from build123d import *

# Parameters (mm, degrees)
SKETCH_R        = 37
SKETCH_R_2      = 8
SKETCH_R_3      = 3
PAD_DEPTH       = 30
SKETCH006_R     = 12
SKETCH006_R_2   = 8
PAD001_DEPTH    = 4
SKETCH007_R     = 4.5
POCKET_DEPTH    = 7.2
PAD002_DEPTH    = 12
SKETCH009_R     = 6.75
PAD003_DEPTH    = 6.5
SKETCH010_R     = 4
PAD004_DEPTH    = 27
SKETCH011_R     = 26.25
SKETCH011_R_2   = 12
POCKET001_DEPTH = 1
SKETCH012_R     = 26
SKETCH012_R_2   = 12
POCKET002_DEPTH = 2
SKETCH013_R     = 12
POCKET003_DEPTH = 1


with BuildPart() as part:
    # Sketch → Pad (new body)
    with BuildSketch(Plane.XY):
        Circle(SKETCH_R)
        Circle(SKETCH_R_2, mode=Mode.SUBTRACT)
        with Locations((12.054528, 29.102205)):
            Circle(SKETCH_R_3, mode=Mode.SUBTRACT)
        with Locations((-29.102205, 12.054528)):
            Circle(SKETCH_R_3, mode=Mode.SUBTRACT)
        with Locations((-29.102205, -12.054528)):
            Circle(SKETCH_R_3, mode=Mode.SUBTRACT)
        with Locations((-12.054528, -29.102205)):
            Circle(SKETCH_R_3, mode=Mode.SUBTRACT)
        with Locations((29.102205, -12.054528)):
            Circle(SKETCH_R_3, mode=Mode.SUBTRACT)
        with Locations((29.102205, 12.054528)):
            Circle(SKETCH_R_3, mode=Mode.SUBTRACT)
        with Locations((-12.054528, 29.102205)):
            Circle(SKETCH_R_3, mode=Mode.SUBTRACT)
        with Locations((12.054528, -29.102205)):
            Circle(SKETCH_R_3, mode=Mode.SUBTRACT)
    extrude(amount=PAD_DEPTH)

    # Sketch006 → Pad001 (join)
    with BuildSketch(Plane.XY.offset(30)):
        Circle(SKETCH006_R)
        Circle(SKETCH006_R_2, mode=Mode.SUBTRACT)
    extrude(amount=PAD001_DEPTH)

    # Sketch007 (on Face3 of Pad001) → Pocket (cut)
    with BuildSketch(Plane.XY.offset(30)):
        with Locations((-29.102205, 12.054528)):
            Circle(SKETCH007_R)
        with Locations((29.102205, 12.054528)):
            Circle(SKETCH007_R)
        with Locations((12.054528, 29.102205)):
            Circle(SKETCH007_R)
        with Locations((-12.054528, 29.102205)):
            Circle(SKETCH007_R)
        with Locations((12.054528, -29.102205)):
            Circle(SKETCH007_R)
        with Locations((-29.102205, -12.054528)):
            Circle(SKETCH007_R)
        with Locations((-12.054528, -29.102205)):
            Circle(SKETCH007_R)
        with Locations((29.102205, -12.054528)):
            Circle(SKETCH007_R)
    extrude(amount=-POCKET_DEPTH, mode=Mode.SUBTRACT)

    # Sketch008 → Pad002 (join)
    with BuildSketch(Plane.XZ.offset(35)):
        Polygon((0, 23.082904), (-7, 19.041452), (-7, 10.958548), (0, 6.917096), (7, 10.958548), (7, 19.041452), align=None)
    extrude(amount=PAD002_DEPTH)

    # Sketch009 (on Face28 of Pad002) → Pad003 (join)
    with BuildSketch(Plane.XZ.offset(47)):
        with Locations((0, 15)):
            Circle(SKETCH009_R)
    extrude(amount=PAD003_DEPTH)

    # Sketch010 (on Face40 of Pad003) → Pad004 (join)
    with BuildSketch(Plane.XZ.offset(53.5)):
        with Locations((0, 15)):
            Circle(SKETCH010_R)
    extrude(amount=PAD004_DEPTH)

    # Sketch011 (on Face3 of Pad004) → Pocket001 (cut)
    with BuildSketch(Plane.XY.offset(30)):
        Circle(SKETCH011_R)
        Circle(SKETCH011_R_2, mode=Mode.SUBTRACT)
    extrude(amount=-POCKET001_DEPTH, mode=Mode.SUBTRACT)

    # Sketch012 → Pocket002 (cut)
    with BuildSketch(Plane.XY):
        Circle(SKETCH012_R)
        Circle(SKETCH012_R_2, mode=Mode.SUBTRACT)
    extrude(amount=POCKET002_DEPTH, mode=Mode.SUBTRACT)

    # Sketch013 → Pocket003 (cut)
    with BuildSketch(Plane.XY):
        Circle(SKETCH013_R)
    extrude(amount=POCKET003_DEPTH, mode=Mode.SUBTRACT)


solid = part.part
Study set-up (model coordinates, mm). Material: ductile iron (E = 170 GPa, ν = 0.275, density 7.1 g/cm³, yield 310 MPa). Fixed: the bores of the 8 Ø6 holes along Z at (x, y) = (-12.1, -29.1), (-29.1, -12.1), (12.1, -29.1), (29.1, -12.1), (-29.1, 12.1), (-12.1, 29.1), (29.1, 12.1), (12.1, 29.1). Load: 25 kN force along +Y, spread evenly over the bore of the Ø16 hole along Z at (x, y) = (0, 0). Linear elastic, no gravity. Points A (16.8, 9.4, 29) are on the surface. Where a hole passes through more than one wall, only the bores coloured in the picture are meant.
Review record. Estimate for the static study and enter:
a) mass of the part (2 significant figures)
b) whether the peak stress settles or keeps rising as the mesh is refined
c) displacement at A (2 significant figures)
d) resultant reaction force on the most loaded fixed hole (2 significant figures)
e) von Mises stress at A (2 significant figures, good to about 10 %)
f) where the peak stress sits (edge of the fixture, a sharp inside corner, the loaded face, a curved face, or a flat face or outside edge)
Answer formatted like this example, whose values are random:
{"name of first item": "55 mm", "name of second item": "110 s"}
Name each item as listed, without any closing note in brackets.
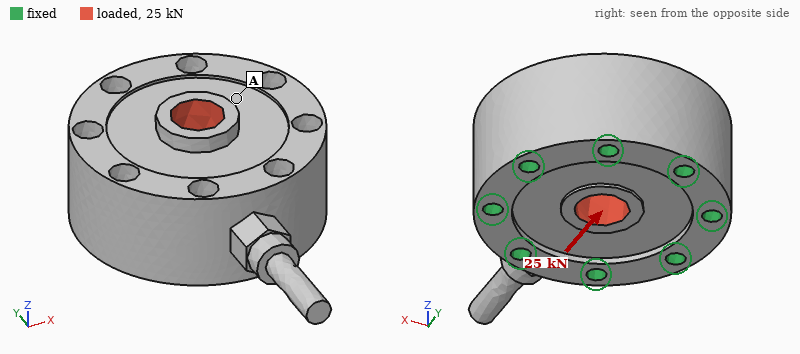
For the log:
{"mass of the part": "810 g", "whether the peak stress settles or keeps rising as the mesh is refined": "keeps rising", "displacement at A": "1.00 µm", "resultant reaction force on the most loaded fixed hole": "4.8 kN", "von Mises stress at A": "7.8 MPa", "where the peak stress sits": "edge of the fixture"}
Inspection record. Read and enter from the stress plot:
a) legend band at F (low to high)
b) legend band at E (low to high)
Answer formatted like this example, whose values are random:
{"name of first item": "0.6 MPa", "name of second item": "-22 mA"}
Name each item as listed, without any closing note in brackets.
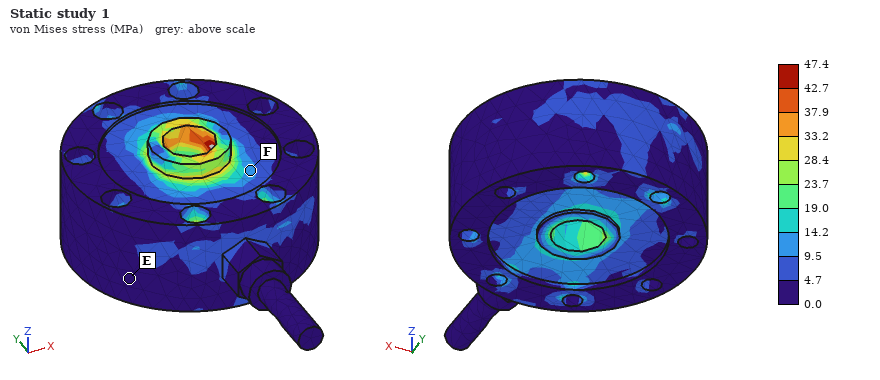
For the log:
{"legend band at F": "9.5 to 14.2 MPa", "legend band at E": "0.0 to 4.7 MPa"}
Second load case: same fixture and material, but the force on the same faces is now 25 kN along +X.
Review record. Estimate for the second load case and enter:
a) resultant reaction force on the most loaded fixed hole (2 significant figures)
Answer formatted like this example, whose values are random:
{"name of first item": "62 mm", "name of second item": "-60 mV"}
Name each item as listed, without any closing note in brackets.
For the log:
{"resultant reaction force on the most loaded fixed hole": "4.8 kN"}
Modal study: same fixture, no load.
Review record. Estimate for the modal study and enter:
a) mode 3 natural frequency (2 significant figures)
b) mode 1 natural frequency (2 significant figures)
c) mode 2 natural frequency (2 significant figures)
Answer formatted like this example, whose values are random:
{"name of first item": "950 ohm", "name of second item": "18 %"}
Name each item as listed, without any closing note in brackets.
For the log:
{"mode 3 natural frequency": "18 kHz", "mode 1 natural frequency": "5300 Hz", "mode 2 natural frequency": "5300 Hz"}
